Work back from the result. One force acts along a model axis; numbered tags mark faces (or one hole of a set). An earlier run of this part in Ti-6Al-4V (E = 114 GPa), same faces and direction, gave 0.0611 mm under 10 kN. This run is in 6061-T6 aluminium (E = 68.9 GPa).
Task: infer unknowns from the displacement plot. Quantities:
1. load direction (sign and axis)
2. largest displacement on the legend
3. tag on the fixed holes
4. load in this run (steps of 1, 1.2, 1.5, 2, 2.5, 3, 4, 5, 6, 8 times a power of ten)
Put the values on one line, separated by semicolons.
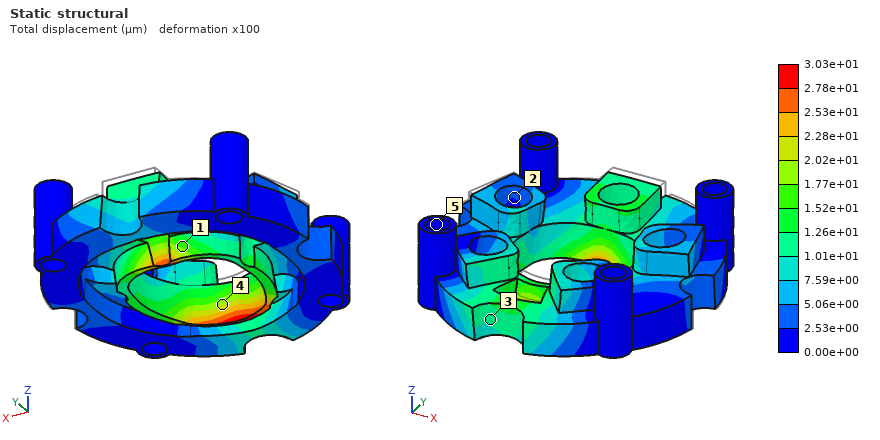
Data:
-Y; 3.03e+01 µm; 5; 3 kN
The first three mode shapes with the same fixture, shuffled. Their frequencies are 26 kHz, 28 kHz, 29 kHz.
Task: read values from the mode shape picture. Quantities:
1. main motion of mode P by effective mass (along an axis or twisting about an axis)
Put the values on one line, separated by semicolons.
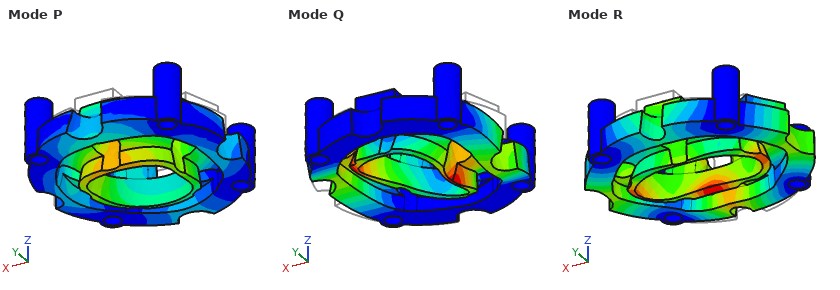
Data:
along Z
